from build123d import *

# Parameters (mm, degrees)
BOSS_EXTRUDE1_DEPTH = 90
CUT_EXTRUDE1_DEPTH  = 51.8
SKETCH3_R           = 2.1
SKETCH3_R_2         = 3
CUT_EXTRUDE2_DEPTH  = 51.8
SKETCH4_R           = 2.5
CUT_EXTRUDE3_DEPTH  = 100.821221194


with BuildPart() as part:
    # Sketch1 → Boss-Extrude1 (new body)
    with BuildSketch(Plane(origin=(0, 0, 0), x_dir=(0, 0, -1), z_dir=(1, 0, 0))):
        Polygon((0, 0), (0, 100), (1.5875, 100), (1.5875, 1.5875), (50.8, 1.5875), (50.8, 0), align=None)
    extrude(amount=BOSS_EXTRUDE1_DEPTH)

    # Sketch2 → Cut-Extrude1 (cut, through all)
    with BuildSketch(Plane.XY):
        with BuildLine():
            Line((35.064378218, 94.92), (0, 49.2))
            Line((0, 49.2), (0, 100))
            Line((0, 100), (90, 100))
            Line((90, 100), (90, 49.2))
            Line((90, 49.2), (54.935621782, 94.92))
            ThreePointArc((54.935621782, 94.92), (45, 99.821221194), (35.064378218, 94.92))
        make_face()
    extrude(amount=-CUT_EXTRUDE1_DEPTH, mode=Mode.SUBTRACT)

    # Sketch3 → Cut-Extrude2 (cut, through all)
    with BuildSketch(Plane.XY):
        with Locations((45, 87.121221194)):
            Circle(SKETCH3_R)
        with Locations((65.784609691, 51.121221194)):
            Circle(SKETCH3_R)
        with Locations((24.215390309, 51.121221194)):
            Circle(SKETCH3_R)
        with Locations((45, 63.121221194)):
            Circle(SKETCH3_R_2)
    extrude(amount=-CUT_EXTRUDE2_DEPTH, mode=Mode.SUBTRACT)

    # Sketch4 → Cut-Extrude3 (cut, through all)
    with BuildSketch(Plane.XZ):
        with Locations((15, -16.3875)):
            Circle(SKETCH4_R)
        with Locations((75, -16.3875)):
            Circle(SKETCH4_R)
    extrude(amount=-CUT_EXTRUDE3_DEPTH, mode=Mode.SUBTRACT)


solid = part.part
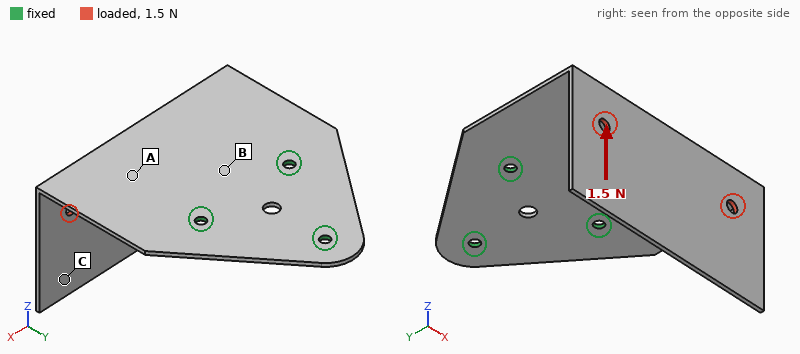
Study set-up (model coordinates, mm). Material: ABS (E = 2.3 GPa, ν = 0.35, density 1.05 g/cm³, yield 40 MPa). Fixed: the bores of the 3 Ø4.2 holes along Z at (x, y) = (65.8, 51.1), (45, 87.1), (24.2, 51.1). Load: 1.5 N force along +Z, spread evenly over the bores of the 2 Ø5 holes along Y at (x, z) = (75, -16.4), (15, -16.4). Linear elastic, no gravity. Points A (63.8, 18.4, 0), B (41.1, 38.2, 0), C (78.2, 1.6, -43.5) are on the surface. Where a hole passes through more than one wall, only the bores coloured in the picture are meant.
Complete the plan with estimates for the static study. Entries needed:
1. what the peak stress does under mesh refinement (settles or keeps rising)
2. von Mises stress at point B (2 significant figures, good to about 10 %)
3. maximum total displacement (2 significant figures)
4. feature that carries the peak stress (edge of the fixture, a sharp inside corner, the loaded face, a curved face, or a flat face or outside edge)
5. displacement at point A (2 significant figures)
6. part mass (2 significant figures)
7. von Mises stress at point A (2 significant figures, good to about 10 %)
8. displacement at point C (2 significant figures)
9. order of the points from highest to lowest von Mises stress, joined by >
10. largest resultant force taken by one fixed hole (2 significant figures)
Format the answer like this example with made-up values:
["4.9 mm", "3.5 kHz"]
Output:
["keeps rising", "1.3 MPa", "1.7 mm", "edge of the fixture", "0.49 mm", "19 g", "0.61 MPa", "1.5 mm", "B > A > C", "0.93 N"]
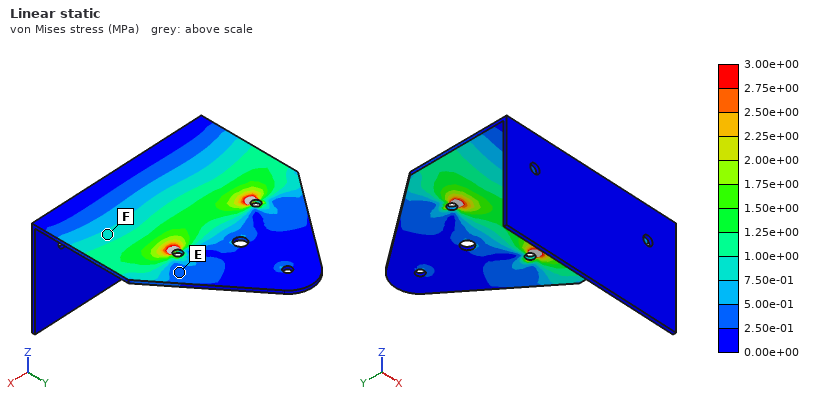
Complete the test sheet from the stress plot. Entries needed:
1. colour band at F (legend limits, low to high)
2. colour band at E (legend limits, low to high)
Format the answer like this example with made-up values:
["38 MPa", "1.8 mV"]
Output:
["7.50e-01 to 1.00e+00 MPa", "2.50e-01 to 5.00e-01 MPa"]
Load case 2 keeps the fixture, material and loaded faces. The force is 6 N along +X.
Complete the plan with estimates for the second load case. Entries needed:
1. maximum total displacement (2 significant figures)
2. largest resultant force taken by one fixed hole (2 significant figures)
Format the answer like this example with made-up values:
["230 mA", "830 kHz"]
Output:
["1.7 mm", "6.9 N"]
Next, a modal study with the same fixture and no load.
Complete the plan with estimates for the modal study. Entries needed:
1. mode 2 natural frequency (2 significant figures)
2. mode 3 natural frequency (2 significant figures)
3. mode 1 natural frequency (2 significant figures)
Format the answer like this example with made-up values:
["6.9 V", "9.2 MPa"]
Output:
["86 Hz", "140 Hz", "50 Hz"]
